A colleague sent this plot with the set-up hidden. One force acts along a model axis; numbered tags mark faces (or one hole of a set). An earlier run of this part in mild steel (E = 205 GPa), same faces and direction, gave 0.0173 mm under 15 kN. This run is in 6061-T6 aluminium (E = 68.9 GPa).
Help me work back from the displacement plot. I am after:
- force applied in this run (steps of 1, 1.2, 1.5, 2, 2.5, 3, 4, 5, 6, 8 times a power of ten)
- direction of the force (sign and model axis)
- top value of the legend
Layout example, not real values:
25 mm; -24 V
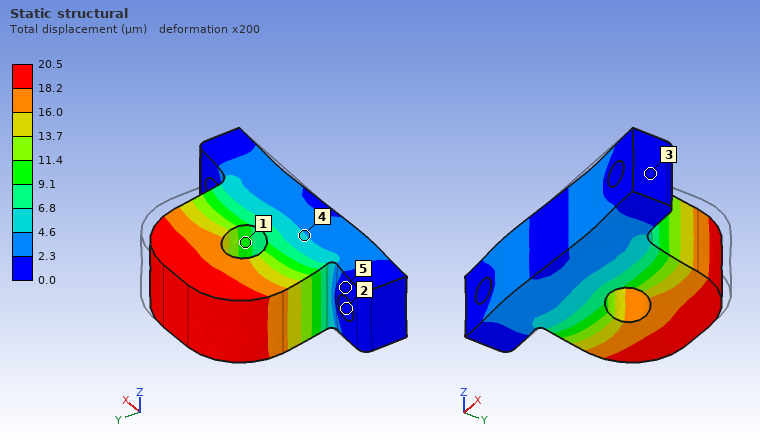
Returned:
6 kN; -X; 20.5 µm
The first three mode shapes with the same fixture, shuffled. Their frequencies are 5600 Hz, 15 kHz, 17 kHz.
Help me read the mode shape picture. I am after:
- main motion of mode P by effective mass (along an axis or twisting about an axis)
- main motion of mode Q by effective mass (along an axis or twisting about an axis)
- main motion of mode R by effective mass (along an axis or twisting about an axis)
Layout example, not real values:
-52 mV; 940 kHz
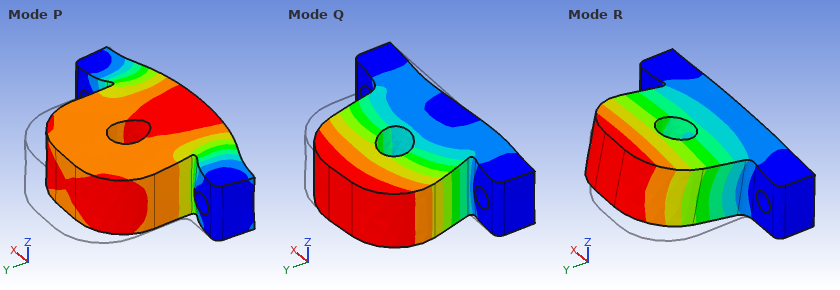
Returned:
along Y; along X; along Z
